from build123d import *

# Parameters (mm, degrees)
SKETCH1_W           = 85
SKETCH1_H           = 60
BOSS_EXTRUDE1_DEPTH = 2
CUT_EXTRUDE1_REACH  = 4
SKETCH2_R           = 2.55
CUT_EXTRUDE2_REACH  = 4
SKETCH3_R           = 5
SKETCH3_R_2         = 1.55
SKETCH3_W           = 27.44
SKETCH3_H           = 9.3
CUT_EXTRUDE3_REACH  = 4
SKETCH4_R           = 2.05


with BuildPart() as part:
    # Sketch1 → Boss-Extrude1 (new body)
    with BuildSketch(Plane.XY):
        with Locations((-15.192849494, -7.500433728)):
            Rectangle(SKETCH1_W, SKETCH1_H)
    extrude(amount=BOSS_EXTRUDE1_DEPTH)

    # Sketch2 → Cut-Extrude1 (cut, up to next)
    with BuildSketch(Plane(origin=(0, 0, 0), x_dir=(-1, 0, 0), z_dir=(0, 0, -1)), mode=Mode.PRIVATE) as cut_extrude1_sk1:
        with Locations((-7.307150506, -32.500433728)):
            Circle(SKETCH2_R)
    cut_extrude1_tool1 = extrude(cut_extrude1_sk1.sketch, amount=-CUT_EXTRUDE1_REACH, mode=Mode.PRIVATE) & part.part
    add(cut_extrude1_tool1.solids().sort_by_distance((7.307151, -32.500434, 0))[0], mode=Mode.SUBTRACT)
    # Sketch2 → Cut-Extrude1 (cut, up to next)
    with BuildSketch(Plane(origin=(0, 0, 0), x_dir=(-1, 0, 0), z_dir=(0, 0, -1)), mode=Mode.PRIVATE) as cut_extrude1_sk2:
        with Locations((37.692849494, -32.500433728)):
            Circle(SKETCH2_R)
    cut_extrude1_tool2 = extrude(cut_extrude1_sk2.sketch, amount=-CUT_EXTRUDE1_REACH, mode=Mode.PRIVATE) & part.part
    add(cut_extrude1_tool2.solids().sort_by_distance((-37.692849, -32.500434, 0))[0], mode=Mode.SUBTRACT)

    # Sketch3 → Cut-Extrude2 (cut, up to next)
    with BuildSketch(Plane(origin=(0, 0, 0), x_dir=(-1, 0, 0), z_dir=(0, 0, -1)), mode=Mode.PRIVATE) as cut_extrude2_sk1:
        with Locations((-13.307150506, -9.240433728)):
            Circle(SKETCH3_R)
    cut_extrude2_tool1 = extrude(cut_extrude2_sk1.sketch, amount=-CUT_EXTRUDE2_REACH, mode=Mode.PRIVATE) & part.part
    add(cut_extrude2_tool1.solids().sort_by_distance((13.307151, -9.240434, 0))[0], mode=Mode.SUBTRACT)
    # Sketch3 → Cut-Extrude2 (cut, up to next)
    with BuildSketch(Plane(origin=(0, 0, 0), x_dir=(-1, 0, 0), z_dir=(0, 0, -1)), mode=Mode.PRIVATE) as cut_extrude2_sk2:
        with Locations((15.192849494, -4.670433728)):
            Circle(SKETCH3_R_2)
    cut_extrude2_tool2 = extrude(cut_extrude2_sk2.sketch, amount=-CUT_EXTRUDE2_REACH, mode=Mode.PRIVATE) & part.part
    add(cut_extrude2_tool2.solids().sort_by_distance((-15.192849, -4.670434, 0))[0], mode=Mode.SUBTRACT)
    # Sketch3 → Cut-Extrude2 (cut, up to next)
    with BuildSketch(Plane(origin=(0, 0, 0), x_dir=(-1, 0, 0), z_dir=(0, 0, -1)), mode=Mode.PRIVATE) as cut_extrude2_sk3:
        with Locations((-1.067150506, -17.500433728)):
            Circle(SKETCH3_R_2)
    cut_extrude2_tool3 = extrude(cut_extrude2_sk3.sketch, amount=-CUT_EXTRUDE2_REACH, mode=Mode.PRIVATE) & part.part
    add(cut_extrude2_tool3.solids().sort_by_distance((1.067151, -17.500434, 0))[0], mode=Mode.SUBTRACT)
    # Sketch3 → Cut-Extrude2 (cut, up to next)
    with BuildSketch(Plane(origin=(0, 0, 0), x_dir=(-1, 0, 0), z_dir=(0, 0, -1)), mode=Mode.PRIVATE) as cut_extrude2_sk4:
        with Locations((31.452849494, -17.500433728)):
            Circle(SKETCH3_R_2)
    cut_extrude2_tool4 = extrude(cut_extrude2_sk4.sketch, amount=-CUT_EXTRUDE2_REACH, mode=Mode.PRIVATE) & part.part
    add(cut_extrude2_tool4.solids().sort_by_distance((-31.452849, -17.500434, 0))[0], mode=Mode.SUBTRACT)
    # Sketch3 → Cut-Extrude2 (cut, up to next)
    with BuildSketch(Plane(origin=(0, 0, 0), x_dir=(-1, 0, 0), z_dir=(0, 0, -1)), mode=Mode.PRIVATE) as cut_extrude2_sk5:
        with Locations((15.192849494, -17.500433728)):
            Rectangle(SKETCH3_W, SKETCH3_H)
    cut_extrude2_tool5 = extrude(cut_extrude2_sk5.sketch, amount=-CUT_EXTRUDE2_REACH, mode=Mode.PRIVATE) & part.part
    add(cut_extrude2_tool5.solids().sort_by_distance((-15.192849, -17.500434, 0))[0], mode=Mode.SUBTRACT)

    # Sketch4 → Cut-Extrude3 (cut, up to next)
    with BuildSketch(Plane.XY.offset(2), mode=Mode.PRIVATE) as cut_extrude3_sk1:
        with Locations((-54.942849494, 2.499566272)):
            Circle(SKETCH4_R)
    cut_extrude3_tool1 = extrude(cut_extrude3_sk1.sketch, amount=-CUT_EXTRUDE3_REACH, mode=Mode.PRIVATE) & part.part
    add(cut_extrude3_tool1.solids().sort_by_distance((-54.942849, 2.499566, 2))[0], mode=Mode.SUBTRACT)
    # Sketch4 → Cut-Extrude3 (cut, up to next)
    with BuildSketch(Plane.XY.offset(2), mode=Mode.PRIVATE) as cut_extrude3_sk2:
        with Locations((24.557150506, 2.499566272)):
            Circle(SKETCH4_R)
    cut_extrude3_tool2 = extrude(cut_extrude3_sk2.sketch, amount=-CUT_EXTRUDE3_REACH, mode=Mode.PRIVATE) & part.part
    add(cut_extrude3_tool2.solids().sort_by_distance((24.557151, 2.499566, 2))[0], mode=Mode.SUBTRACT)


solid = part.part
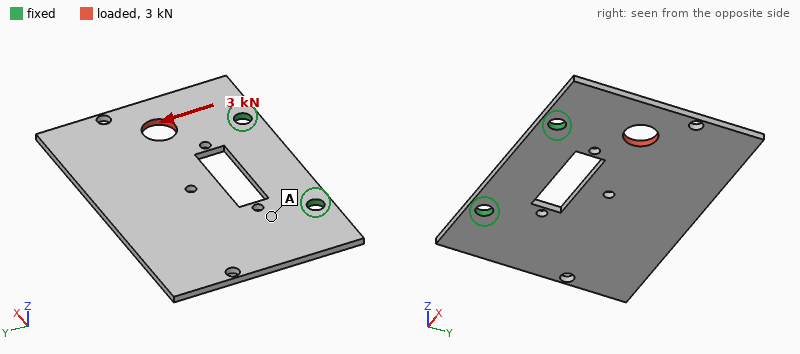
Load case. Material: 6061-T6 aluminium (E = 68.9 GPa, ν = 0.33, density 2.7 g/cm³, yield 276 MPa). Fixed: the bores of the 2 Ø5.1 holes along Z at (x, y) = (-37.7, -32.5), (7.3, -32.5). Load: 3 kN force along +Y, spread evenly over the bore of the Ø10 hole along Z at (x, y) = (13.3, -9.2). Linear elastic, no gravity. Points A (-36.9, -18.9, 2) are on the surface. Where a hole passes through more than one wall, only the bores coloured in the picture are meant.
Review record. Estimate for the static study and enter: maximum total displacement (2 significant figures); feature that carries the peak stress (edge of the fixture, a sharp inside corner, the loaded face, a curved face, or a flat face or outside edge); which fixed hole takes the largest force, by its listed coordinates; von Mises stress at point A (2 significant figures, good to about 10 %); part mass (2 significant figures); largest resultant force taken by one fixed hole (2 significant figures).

74 µm
edge of the fixture
(7.3, -32.5)
16 MPa
25 g
3.2 kN
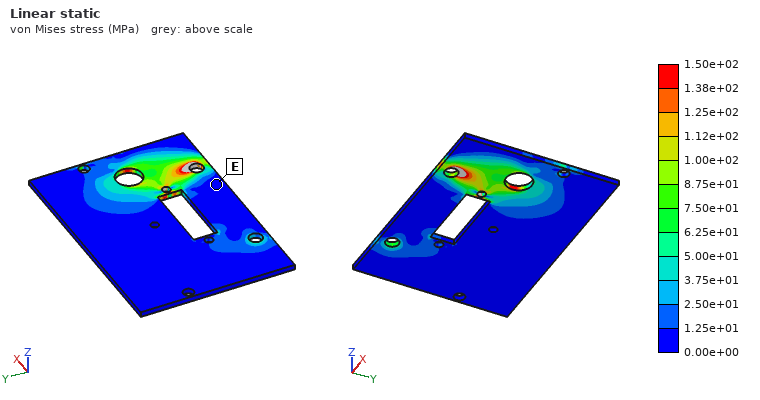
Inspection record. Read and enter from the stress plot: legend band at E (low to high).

0.00e+00 to 1.25e+01 MPa
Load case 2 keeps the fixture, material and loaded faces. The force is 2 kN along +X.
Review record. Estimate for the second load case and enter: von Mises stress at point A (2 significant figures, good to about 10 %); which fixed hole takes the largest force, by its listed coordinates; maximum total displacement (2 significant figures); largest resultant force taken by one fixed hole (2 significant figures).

55 MPa
(7.3, -32.5)
74 µm
1.4 kN
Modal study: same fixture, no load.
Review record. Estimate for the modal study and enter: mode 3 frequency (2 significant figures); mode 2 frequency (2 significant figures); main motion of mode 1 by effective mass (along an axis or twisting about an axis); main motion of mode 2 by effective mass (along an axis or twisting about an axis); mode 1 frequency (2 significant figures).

1900 Hz
880 Hz
along Z
twisting about Y
440 Hz
